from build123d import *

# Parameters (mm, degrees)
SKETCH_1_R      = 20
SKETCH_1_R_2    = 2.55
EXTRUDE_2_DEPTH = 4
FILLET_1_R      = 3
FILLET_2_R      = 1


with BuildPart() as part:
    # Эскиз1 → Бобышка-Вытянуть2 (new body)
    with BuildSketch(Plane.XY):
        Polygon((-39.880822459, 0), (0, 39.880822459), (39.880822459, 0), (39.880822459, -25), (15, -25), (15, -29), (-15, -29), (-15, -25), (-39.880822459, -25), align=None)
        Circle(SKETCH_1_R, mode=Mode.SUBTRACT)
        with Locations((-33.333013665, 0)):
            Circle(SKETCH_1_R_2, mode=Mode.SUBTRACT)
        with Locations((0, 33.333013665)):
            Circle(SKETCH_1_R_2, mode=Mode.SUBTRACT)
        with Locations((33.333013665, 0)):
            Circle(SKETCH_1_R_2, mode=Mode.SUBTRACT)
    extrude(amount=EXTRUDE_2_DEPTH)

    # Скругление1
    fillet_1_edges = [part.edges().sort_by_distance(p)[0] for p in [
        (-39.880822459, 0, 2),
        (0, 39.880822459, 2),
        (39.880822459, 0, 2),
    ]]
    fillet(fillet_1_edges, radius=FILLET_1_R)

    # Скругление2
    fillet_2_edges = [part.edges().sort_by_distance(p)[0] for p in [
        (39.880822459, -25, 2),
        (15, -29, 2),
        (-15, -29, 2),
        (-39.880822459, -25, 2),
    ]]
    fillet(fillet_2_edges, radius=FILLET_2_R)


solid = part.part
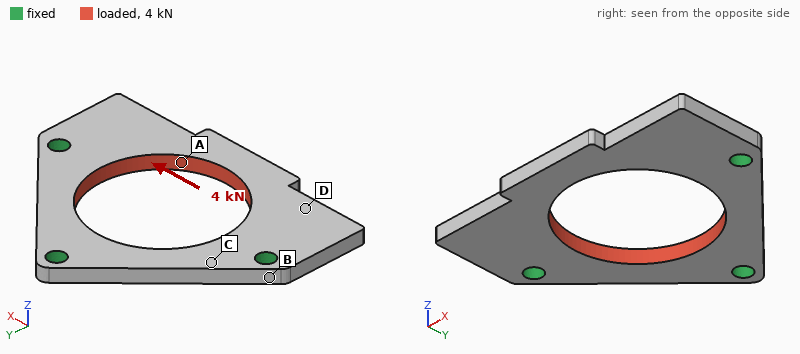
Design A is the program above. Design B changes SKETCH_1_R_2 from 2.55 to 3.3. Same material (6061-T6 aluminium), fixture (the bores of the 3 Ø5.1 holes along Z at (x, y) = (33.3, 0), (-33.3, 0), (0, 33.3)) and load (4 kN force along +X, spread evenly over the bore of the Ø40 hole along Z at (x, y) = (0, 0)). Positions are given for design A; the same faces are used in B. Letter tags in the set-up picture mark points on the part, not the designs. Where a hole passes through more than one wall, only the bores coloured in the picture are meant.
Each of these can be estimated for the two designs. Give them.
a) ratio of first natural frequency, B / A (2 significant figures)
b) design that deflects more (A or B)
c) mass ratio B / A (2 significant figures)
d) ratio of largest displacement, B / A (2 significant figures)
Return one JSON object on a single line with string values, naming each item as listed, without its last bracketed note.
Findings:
{"ratio of first natural frequency, B / A": "1.1", "design that deflects more": "A", "mass ratio B / A": "0.98", "ratio of largest displacement, B / A": "0.91"}
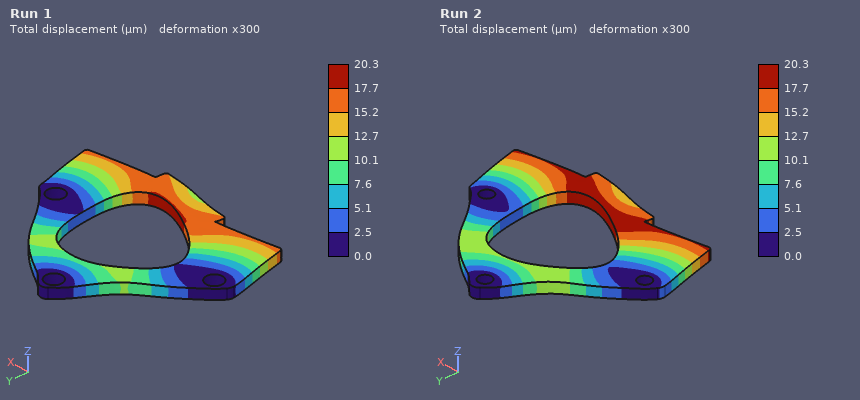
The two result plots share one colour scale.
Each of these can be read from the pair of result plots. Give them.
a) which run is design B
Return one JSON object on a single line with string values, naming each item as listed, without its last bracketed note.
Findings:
{"which run is design B": "Run 1"}
